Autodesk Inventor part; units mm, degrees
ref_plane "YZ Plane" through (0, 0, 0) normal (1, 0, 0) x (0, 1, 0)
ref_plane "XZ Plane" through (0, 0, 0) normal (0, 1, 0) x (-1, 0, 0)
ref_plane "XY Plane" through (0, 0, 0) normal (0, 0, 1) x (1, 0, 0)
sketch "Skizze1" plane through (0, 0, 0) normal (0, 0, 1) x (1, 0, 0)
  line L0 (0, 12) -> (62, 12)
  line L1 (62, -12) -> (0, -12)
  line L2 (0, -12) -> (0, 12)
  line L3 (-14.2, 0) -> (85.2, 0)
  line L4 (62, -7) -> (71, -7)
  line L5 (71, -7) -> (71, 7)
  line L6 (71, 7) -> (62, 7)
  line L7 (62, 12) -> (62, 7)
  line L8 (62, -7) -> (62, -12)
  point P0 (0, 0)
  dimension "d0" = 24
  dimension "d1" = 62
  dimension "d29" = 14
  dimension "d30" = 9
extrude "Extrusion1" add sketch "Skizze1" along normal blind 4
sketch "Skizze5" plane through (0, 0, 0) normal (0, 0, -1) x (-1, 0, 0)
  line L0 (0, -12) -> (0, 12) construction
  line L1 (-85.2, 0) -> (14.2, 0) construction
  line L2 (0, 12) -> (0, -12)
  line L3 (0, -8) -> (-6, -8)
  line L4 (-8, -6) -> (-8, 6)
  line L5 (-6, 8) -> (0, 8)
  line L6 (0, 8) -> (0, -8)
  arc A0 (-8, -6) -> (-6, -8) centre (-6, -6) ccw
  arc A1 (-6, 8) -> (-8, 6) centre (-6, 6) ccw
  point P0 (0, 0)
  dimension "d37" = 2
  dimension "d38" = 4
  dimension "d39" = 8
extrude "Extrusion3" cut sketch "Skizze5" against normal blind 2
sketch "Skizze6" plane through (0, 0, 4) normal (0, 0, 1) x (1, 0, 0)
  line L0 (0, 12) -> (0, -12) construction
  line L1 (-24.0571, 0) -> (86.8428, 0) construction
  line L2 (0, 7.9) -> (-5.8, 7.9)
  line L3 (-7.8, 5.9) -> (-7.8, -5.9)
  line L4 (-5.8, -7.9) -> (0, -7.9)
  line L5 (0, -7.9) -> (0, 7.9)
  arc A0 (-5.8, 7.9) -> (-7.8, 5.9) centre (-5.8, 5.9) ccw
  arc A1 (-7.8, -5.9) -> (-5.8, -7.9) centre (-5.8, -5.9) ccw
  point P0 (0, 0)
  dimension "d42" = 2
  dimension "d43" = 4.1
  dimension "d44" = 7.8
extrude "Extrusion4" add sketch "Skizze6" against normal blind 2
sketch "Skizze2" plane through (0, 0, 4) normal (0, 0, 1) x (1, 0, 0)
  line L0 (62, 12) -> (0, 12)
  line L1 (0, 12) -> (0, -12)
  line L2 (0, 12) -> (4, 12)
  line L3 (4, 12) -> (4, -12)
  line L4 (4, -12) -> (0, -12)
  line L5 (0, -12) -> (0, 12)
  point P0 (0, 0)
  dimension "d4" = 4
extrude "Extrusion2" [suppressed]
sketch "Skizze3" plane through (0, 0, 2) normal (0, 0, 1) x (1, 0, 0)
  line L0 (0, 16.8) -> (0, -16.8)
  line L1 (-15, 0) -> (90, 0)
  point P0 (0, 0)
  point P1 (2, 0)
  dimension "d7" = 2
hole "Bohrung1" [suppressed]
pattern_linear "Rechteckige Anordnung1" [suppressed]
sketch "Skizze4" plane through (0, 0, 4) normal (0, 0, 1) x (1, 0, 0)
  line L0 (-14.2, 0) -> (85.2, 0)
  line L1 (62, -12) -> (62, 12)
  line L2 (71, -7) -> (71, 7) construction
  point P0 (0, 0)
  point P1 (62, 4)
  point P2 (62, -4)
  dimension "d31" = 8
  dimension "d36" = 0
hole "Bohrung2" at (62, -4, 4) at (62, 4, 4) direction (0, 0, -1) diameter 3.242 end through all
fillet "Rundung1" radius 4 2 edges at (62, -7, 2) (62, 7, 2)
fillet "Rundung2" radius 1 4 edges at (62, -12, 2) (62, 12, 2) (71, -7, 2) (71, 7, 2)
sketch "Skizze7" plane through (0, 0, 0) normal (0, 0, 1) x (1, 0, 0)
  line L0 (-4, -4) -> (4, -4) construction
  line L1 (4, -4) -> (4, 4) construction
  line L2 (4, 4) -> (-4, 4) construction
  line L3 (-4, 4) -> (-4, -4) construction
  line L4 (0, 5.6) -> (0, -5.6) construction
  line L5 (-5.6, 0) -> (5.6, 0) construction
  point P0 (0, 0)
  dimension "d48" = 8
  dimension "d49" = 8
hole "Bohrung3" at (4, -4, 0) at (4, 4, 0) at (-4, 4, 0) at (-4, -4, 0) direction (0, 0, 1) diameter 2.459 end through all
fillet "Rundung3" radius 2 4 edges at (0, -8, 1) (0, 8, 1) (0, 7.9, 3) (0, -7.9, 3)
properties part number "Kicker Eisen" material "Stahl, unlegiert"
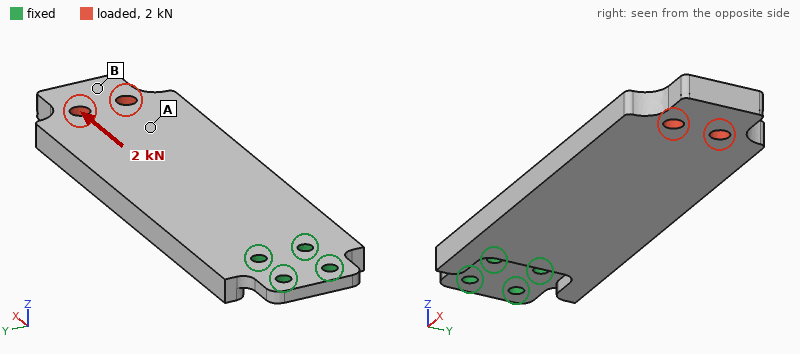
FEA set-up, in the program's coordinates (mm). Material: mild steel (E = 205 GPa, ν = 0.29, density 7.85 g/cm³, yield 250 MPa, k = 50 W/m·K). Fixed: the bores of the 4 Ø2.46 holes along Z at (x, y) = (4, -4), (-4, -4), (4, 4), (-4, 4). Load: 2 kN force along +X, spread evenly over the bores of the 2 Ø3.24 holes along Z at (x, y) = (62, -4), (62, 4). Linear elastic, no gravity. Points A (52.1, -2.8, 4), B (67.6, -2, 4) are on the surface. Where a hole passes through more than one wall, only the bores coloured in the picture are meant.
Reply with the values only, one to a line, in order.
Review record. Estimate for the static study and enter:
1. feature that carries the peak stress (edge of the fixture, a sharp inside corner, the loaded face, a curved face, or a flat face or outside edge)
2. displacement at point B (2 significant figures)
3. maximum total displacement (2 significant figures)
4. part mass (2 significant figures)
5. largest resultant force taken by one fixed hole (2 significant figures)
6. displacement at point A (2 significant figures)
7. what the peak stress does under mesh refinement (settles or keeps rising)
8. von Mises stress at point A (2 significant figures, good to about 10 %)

edge of the fixture
88 µm
93 µm
50 g
810 N
66 µm
keeps rising
26 MPa
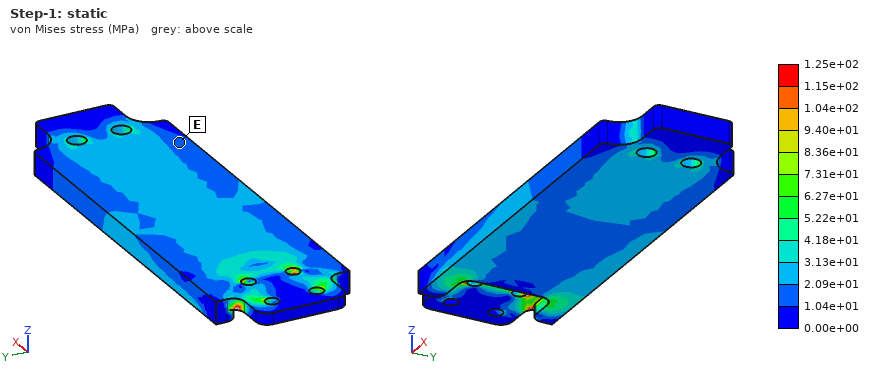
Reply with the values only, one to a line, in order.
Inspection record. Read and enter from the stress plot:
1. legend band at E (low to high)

1.04e+01 to 2.09e+01 MPa
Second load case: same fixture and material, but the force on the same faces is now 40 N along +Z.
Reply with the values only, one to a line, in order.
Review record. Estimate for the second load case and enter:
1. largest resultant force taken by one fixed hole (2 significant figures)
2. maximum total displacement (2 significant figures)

100 N
0.21 mm
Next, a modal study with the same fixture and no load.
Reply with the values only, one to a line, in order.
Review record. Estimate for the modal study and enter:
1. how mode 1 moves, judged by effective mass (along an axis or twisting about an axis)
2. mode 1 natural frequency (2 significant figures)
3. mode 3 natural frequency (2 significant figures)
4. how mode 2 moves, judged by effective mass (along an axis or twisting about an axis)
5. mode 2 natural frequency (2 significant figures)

along Z
600 Hz
3800 Hz
along Y
3100 Hz
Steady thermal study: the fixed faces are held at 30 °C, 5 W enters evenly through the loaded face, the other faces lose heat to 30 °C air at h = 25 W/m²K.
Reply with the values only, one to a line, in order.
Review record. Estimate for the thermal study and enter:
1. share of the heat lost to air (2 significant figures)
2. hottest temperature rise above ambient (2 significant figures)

45 %
48 K
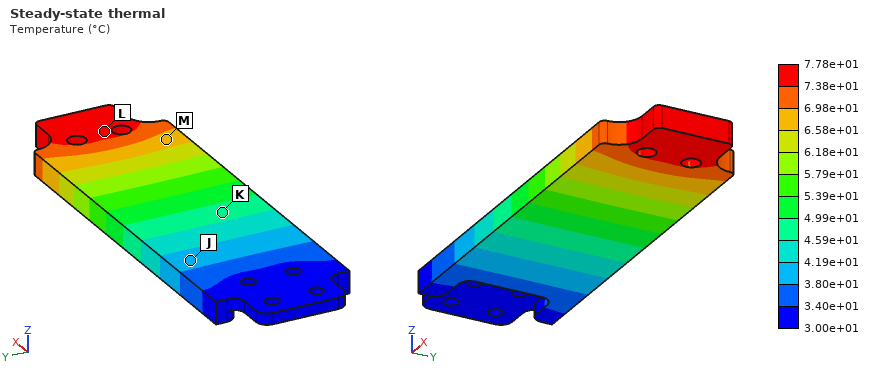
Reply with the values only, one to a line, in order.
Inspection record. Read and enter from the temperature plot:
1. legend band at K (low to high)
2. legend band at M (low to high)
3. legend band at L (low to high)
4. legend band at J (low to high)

4.59e+01 to 4.99e+01 °C
6.58e+01 to 6.98e+01 °C
7.38e+01 to 7.78e+01 °C
3.80e+01 to 4.19e+01 °C
